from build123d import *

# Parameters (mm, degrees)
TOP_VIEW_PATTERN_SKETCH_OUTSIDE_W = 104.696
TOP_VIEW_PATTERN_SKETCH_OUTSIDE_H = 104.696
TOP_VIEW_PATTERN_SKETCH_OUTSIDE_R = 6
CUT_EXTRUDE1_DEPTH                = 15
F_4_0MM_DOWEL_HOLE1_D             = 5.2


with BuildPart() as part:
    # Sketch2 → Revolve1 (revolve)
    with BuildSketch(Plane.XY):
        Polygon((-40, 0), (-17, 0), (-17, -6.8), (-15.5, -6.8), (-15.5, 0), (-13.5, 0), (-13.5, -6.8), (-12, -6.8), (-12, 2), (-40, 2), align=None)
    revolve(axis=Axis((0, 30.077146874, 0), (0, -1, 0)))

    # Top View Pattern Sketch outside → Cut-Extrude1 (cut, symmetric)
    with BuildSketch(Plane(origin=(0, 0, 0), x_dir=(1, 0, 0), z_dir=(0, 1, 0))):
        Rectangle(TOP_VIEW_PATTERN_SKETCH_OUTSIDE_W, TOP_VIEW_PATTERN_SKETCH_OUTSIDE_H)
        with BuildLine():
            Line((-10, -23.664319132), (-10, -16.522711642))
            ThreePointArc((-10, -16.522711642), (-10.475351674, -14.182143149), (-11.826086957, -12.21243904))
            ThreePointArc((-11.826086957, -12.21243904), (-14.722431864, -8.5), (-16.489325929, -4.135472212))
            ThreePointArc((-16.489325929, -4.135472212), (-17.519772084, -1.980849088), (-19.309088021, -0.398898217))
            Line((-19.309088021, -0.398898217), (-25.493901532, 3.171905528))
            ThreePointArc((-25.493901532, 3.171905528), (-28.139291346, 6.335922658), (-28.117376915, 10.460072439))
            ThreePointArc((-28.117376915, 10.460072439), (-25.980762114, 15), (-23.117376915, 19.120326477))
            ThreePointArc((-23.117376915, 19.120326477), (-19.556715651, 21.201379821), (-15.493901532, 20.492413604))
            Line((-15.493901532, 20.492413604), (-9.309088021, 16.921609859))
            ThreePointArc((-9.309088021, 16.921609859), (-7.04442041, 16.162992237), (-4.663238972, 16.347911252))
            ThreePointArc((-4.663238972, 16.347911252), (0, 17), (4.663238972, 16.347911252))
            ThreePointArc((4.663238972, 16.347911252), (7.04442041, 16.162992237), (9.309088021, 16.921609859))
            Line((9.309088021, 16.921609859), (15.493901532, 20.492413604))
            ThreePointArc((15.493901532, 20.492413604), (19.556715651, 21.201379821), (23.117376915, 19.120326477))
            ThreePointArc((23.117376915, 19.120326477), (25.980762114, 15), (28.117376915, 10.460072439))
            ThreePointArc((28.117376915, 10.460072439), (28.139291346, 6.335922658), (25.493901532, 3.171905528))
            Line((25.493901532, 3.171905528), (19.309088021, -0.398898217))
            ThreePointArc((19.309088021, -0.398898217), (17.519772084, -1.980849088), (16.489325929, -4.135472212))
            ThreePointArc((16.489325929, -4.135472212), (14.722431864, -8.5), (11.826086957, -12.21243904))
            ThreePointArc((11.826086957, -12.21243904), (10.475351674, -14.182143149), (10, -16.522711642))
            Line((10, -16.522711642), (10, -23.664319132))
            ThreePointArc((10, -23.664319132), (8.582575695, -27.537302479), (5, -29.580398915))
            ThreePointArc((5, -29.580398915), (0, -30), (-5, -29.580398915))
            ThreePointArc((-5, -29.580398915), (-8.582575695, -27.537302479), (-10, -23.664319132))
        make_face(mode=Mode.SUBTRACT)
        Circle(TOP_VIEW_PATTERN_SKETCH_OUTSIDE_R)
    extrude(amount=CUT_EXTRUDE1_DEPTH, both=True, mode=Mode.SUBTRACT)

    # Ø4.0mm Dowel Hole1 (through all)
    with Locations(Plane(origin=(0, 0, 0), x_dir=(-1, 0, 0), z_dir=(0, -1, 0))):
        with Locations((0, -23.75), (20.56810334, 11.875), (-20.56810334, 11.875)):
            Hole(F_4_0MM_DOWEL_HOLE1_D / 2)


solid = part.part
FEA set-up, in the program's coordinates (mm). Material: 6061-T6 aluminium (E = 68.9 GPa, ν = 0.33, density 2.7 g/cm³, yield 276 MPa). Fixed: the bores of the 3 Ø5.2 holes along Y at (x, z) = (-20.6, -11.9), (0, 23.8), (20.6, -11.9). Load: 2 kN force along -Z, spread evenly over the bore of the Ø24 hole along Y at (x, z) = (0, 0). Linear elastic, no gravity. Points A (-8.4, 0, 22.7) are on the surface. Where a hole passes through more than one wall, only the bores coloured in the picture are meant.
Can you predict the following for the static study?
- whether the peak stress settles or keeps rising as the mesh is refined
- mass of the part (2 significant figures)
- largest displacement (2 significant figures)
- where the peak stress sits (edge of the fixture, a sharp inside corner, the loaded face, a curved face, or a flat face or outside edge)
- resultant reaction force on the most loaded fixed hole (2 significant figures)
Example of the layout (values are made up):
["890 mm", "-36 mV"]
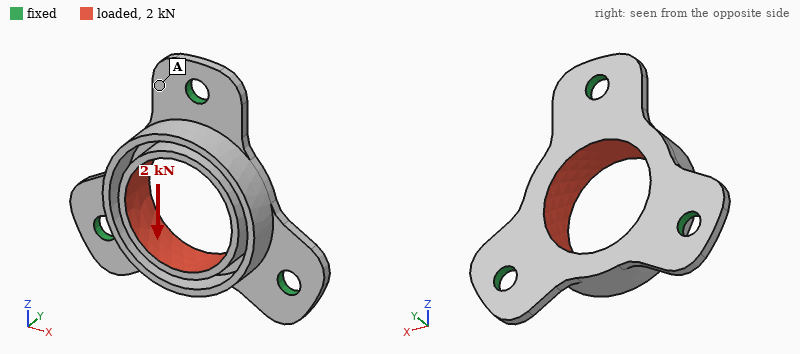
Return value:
["keeps rising", "11 g", "68 µm", "edge of the fixture", "680 N"]
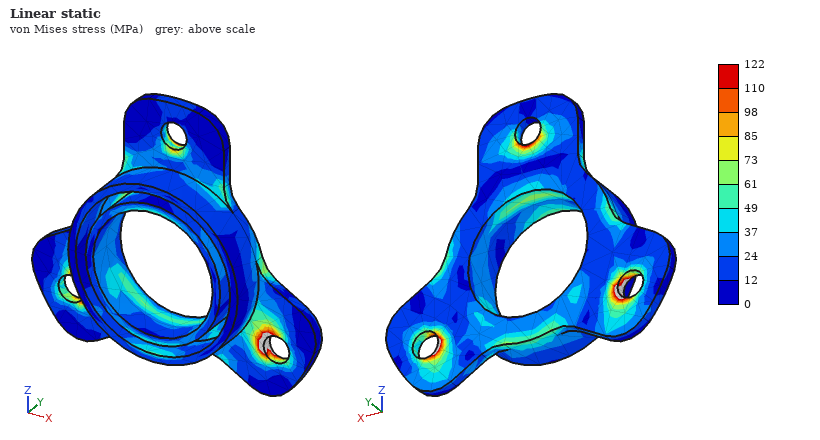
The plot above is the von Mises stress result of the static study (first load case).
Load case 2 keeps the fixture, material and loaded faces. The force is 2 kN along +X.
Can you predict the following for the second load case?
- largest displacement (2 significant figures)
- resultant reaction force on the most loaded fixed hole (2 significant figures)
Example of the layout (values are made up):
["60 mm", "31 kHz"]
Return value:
["60 µm", "680 N"]
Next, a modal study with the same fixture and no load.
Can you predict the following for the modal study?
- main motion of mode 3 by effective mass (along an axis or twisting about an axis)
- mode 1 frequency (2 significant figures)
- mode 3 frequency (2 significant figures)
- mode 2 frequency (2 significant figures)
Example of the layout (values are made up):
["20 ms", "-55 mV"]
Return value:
["along Y", "8800 Hz", "9500 Hz", "8800 Hz"]
